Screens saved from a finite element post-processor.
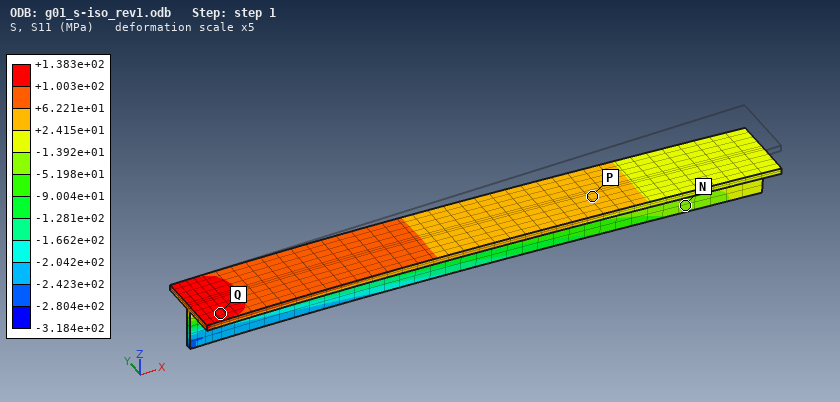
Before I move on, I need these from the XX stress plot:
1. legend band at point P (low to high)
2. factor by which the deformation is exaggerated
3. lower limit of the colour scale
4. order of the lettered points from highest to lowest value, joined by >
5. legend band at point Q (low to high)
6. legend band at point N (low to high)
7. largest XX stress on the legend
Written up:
+2.415e+01 to +6.221e+01 MPa
5
-3.184e+02 MPa
Q > P > N
+1.003e+02 to +1.383e+02 MPa
-5.198e+01 to -1.392e+01 MPa
+1.383e+02 MPa
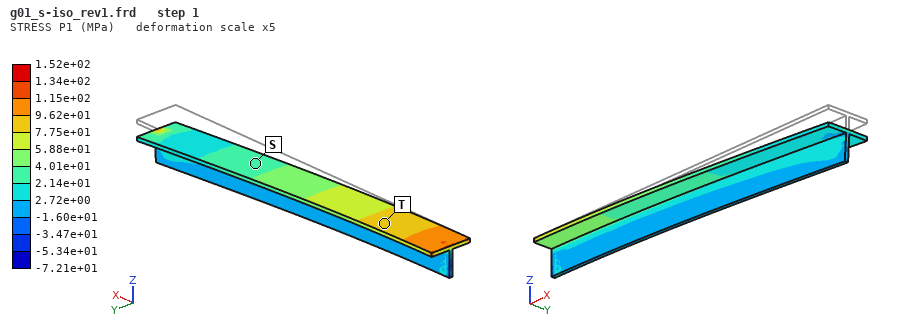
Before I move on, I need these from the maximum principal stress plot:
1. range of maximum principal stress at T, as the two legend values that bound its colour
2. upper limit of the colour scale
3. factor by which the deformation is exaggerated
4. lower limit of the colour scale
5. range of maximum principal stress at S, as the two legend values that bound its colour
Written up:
7.75e+01 to 9.62e+01 MPa
1.52e+02 MPa
5
-7.21e+01 MPa
2.14e+01 to 4.01e+01 MPa
